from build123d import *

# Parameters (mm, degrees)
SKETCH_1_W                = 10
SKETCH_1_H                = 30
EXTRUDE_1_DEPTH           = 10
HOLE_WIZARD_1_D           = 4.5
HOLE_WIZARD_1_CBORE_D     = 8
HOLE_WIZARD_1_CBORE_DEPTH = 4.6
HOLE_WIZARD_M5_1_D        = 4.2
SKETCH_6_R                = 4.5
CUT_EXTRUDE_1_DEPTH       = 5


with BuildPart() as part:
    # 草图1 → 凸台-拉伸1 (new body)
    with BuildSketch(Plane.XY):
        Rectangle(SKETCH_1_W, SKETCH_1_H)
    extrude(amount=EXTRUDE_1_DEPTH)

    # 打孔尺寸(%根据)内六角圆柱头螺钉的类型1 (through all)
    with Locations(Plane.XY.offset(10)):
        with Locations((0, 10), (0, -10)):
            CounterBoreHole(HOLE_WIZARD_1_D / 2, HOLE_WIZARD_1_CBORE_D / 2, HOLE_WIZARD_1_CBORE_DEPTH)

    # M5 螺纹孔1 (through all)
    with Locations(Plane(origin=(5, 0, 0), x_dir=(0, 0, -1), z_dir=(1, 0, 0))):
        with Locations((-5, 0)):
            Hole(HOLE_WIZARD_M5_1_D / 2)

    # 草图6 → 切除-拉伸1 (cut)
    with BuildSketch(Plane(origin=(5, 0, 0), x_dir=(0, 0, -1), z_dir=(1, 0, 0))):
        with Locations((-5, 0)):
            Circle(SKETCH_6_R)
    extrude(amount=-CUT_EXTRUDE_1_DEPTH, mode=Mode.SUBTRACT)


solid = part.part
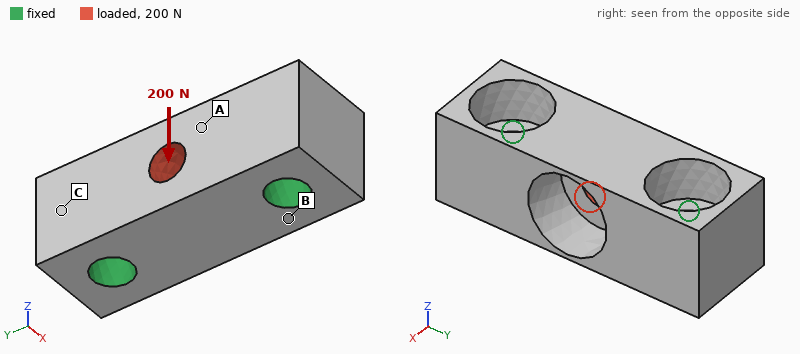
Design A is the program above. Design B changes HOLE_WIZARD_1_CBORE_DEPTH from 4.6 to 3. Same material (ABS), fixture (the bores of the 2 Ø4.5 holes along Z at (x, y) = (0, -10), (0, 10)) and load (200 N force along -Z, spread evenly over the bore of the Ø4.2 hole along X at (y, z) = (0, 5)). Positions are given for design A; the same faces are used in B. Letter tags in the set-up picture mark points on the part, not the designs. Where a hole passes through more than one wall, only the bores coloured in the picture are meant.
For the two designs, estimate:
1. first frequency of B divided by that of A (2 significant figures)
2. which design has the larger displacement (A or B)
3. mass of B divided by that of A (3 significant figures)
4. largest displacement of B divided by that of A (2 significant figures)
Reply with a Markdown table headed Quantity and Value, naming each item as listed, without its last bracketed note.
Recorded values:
| Quantity | Value |
|---|---|
| first frequency of B divided by that of A | 1.3 |
| which design has the larger displacement | A |
| mass of B divided by that of A | 1.06 |
| largest displacement of B divided by that of A | 0.83 |
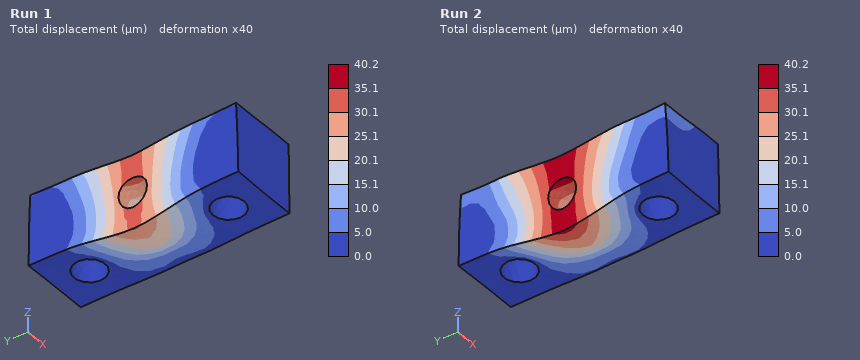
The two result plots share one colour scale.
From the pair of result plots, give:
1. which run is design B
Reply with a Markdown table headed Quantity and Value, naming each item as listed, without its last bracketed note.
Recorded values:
| Quantity | Value |
|---|---|
| which run is design B | Run 1 |
